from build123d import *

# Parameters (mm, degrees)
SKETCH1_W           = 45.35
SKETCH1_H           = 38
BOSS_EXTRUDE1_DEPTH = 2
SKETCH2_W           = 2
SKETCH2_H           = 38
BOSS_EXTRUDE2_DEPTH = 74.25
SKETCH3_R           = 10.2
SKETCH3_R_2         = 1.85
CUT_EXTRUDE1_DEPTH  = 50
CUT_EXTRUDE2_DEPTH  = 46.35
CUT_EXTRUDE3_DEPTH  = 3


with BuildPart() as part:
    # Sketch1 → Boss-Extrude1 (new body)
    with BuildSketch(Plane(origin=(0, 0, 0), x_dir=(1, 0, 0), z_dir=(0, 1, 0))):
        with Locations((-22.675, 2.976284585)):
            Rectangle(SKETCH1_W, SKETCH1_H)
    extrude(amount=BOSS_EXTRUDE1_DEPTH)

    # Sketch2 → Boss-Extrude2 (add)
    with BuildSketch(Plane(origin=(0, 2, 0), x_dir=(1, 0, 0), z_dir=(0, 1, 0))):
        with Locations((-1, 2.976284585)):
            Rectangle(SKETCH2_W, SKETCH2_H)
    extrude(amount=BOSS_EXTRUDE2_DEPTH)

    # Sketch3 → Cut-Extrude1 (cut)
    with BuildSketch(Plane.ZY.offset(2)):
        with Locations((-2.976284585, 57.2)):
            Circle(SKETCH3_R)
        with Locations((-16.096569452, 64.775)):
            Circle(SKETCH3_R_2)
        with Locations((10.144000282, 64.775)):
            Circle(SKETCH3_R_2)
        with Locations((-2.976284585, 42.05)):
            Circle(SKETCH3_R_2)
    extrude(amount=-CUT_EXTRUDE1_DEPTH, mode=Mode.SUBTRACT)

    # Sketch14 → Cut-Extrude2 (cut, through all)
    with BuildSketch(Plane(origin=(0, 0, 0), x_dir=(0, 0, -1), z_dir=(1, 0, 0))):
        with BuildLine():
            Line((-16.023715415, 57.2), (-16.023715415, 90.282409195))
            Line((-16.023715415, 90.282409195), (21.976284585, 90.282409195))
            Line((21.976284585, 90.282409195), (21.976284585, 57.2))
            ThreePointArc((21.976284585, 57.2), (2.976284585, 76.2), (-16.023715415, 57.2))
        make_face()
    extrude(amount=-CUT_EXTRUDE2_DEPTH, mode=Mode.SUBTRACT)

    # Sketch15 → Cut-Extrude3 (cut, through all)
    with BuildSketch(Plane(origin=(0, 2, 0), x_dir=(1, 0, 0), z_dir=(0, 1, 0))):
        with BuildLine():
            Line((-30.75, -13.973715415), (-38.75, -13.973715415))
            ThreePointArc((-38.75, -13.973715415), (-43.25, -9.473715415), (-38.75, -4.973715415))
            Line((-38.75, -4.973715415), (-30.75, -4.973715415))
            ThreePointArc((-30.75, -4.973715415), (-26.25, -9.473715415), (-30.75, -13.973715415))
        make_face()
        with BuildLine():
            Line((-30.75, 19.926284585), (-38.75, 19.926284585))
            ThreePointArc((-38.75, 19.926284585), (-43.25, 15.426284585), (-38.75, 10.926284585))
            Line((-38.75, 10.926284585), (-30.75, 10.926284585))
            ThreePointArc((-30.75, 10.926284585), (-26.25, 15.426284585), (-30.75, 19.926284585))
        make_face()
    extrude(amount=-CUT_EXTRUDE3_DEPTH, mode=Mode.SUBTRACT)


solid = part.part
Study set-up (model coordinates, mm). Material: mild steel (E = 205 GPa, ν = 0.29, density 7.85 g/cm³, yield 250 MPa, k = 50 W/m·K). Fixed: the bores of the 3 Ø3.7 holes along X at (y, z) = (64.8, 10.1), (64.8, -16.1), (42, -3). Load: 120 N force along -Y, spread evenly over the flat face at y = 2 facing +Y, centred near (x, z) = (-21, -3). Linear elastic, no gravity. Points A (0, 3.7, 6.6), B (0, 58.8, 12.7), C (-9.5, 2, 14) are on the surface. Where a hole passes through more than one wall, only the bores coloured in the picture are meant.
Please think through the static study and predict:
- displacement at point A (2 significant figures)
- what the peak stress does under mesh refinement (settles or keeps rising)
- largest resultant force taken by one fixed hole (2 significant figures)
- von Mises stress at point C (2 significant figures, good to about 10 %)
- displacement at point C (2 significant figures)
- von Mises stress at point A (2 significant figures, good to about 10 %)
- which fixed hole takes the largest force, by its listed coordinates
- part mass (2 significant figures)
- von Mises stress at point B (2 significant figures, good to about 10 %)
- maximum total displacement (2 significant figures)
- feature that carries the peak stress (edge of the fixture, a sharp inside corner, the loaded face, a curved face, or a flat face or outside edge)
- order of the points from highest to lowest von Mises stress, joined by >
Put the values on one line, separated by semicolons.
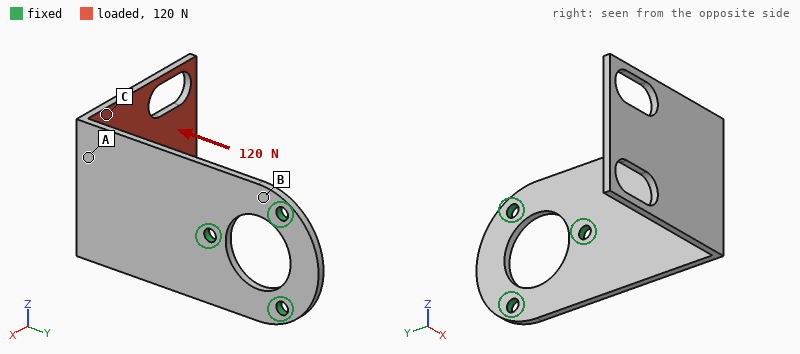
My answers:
0.35 mm; keeps rising; 97 N; 56 MPa; 0.42 mm; 84 MPa; (42, -3); 59 g; 14 MPa; 1.1 mm; edge of the fixture; A > C > B
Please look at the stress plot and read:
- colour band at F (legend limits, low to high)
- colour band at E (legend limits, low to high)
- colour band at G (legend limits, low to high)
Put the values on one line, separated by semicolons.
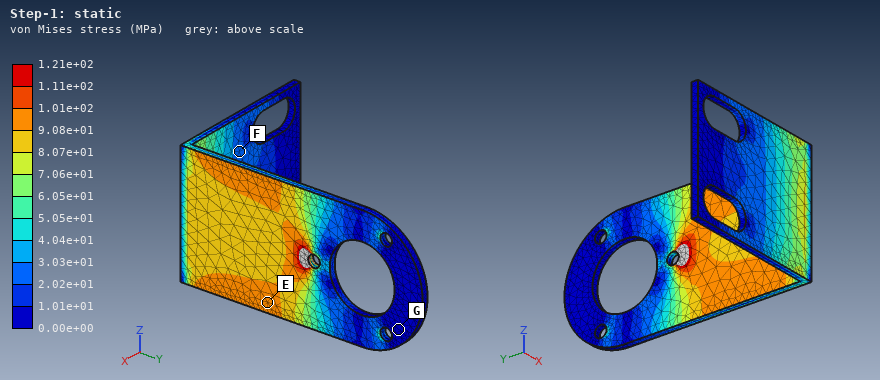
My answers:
2.02e+01 to 3.03e+01 MPa; 9.08e+01 to 1.01e+02 MPa; 0.00e+00 to 1.01e+01 MPa
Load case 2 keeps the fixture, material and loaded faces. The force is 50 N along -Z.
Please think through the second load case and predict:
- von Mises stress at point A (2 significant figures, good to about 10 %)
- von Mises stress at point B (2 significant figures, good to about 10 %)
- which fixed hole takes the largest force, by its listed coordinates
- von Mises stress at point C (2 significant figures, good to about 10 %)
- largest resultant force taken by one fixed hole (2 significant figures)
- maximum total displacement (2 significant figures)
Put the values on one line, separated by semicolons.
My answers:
24 MPa; 18 MPa; (42, -3); 14 MPa; 66 N; 0.25 mm
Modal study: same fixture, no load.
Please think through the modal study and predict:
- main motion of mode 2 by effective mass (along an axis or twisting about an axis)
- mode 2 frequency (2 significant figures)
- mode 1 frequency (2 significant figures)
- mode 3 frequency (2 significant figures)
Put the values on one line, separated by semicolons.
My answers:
along Z; 560 Hz; 340 Hz; 920 Hz
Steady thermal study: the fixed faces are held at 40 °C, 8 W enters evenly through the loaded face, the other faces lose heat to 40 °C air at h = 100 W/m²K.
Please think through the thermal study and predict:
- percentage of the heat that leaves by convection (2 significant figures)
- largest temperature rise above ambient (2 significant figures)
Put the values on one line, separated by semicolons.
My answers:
92 %; 31 K
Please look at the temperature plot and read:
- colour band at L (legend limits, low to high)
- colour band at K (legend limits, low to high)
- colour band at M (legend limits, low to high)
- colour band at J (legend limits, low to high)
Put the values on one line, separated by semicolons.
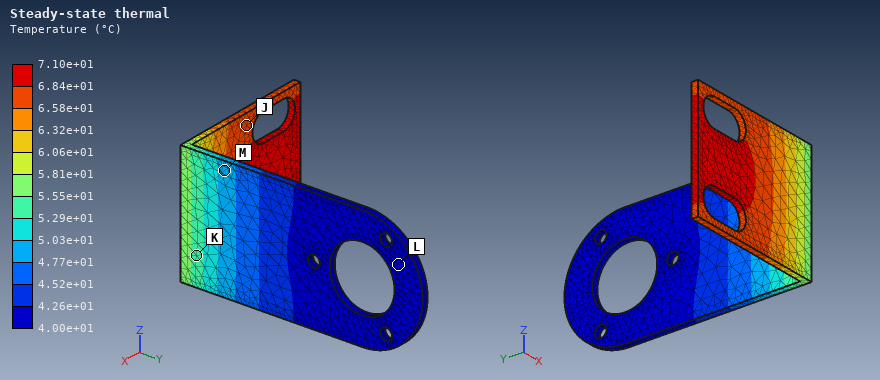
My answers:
4.00e+01 to 4.26e+01 °C; 5.29e+01 to 5.55e+01 °C; 4.77e+01 to 5.03e+01 °C; 6.58e+01 to 6.84e+01 °C
